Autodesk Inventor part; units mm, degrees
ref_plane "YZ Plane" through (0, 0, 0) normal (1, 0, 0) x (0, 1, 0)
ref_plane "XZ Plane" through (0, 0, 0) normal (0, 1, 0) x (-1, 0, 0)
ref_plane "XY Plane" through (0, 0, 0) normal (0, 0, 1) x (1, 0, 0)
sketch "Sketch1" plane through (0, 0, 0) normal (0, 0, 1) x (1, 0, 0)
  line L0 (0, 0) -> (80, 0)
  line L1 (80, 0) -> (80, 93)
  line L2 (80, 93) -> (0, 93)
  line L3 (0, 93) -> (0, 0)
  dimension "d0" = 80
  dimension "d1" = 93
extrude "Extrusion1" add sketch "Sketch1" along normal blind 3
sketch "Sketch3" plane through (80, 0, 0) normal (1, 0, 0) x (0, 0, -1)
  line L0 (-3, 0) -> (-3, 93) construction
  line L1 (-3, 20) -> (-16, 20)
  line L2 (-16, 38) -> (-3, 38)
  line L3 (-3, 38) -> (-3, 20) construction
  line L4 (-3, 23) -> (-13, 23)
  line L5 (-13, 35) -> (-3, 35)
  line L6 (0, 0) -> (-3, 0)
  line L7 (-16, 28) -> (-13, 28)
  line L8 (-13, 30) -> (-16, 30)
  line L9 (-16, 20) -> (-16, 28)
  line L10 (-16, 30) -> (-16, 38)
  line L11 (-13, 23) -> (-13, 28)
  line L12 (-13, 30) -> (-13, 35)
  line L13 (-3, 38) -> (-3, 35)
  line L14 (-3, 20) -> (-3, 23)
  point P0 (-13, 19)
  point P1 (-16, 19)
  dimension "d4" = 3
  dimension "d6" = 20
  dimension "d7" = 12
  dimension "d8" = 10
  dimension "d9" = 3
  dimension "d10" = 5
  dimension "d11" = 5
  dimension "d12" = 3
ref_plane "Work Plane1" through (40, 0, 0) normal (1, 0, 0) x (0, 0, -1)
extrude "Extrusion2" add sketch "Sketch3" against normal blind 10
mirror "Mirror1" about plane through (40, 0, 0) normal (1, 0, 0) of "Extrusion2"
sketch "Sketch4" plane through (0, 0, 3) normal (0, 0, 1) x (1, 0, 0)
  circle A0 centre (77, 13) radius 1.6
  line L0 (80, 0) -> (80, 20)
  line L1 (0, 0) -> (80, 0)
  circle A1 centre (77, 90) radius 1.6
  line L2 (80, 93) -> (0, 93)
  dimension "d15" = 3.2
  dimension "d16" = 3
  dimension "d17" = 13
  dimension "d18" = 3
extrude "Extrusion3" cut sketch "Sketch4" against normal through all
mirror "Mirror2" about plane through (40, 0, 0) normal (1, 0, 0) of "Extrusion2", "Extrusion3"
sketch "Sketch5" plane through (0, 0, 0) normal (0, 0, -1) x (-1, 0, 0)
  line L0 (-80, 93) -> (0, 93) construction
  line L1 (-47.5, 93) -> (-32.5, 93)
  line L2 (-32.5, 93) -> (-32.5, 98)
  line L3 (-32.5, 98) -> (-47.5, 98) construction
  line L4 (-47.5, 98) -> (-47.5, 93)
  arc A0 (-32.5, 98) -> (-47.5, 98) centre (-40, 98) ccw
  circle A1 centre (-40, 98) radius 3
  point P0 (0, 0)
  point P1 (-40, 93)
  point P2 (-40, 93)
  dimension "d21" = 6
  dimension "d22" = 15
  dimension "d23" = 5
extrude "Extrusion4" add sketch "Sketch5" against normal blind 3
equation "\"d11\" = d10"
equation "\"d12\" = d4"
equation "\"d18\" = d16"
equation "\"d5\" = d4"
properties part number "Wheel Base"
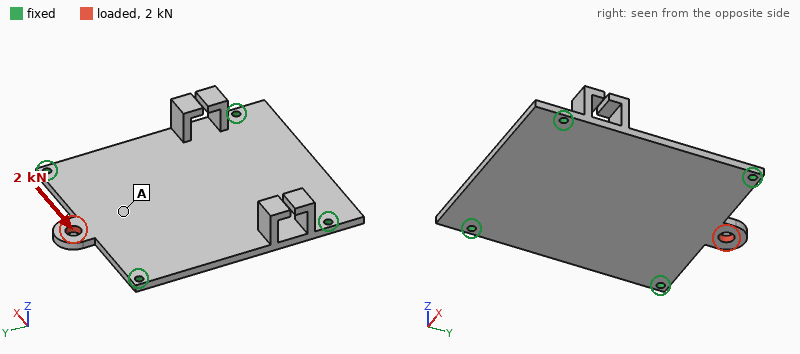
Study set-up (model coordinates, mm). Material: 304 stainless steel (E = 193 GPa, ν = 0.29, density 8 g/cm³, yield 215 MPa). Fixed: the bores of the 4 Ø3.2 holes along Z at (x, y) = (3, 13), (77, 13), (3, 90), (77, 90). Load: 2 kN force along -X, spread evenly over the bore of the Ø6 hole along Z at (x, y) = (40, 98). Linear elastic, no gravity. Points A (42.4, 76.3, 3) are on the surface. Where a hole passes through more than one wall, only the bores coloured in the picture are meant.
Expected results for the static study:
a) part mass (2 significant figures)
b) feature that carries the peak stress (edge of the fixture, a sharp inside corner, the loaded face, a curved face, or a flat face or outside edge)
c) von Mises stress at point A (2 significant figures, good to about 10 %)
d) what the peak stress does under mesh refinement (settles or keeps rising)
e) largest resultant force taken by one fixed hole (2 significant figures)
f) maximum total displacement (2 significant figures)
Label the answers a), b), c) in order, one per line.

a) 200 g
b) a sharp inside corner
c) 13 MPa
d) keeps rising
e) 890 N
f) 24 µm
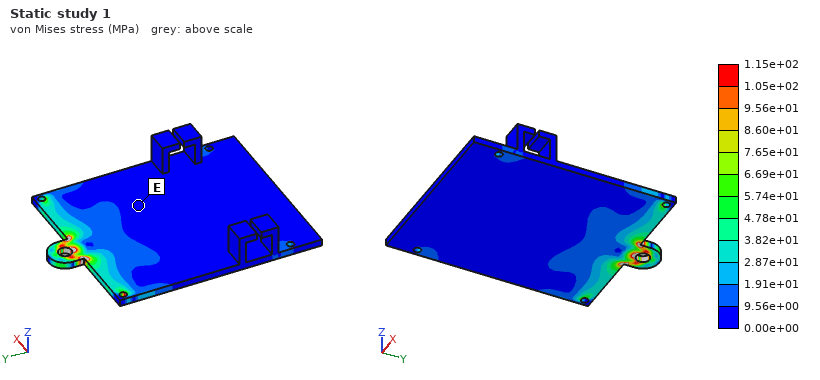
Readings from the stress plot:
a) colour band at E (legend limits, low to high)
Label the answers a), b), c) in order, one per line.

a) 0.00e+00 to 9.56e+00 MPa
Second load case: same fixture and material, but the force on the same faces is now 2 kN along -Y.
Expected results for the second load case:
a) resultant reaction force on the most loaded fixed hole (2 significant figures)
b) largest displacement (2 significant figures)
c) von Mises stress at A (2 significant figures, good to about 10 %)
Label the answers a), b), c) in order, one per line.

a) 540 N
b) 9.6 µm
c) 22 MPa
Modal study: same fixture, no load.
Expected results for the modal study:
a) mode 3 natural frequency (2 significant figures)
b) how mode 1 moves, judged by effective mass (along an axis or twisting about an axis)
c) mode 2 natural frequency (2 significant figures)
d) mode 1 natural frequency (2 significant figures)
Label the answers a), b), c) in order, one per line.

a) 2600 Hz
b) along Z
c) 2500 Hz
d) 1500 Hz
